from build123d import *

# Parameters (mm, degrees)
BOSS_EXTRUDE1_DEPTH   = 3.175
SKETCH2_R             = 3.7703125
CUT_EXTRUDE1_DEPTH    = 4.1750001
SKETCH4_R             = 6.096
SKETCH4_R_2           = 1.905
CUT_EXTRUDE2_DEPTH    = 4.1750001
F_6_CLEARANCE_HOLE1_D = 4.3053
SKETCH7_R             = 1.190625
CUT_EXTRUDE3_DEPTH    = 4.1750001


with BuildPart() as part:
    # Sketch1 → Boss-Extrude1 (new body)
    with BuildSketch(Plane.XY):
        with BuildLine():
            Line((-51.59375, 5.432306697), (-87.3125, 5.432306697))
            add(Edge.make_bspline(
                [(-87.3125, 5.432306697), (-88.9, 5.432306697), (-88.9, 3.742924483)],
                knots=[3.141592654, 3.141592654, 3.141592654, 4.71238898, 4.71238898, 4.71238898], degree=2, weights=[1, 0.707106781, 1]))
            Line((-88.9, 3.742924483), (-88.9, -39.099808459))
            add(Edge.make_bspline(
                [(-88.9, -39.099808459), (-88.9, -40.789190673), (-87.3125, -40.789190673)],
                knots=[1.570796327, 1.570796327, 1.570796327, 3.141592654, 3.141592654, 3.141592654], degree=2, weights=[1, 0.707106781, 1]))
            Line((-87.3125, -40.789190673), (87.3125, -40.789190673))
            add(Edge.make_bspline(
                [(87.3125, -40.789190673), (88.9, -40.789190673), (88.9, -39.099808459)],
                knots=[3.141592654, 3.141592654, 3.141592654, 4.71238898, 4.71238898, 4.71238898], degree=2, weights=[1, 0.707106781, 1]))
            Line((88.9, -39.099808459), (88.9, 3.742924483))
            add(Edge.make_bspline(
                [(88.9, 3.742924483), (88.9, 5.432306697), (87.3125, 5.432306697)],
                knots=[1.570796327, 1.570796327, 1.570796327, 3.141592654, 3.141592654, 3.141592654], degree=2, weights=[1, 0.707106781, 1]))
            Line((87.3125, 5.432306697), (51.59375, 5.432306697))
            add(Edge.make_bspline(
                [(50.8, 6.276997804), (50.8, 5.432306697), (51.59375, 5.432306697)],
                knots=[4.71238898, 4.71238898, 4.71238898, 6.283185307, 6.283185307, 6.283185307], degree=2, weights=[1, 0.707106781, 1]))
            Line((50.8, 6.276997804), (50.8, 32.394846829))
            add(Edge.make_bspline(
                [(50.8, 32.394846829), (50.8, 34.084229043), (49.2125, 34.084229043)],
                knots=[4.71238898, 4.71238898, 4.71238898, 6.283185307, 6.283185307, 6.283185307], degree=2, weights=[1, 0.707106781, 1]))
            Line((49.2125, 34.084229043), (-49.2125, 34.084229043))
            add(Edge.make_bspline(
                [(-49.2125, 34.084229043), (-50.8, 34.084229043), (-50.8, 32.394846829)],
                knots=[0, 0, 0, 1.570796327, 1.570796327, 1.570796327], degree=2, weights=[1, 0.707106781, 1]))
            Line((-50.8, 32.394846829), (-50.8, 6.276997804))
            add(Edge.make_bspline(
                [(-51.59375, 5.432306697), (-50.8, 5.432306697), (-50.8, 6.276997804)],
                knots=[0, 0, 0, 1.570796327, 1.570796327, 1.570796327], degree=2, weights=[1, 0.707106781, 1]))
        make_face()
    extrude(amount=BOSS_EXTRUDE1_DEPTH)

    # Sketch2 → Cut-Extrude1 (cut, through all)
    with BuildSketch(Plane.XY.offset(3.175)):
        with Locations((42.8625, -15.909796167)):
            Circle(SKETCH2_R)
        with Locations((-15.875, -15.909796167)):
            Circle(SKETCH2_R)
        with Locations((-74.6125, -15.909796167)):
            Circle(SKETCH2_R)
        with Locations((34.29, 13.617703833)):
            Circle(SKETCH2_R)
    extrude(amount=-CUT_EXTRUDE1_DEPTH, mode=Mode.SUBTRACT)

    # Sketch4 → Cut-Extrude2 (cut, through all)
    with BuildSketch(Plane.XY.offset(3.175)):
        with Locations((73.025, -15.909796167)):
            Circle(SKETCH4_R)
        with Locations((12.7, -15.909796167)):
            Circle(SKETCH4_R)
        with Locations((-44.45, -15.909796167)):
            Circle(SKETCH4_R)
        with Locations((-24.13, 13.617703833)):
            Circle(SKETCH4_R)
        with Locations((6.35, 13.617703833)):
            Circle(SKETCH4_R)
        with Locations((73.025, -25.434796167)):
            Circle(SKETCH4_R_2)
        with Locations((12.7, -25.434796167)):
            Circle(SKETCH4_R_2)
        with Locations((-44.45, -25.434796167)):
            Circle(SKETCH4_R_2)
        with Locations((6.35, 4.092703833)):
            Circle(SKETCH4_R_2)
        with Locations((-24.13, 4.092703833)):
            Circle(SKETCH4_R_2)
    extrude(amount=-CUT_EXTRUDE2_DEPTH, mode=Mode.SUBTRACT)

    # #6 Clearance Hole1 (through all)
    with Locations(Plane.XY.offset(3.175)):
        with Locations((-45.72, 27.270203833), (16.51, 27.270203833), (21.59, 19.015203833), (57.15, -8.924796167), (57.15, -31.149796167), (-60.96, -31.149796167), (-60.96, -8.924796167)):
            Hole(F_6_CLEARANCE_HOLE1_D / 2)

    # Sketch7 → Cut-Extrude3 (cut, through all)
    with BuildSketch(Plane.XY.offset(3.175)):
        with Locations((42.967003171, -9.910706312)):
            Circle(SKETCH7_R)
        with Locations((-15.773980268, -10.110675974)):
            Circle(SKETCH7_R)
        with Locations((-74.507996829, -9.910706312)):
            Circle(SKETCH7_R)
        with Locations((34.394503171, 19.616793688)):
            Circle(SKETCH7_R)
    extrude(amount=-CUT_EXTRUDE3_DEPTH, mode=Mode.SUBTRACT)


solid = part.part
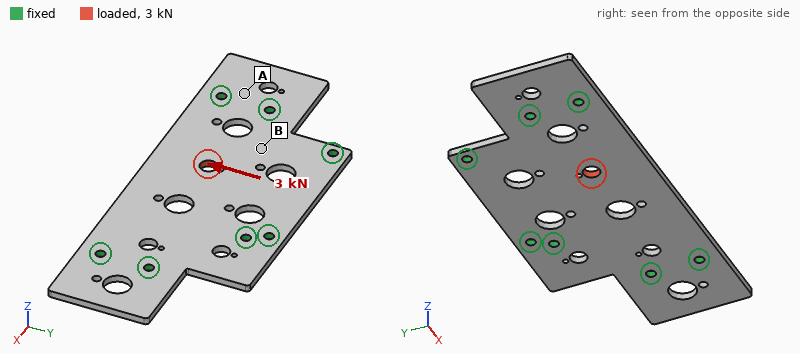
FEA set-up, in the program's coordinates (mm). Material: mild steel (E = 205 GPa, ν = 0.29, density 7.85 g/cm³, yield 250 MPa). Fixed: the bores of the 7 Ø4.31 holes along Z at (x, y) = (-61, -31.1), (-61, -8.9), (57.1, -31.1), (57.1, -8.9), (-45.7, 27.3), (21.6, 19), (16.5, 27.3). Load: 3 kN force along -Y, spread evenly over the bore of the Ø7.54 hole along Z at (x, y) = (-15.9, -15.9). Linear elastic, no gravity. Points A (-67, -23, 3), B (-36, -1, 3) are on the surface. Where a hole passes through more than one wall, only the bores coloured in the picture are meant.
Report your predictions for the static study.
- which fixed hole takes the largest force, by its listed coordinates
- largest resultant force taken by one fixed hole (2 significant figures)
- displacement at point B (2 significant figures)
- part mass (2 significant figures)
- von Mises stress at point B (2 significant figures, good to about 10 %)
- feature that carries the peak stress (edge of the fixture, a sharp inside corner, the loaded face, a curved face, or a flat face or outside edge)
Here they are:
(-45.7, 27.3)
1.1 kN
3.0 µm
250 g
17 MPa
a curved face
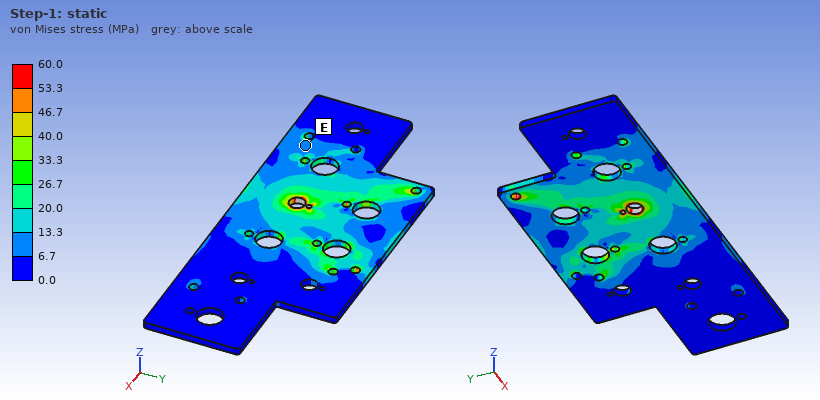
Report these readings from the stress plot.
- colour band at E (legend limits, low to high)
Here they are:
6.7 to 13.3 MPa
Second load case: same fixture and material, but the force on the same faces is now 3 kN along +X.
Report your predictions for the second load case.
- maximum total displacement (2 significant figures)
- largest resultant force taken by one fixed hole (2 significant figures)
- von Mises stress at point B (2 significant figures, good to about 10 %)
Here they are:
4.7 µm
730 N
9.9 MPa
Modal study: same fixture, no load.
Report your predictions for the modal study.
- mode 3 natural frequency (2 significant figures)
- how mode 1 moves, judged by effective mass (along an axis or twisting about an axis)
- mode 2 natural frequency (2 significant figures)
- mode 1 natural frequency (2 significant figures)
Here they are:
3300 Hz
along Z
2500 Hz
1500 Hz
